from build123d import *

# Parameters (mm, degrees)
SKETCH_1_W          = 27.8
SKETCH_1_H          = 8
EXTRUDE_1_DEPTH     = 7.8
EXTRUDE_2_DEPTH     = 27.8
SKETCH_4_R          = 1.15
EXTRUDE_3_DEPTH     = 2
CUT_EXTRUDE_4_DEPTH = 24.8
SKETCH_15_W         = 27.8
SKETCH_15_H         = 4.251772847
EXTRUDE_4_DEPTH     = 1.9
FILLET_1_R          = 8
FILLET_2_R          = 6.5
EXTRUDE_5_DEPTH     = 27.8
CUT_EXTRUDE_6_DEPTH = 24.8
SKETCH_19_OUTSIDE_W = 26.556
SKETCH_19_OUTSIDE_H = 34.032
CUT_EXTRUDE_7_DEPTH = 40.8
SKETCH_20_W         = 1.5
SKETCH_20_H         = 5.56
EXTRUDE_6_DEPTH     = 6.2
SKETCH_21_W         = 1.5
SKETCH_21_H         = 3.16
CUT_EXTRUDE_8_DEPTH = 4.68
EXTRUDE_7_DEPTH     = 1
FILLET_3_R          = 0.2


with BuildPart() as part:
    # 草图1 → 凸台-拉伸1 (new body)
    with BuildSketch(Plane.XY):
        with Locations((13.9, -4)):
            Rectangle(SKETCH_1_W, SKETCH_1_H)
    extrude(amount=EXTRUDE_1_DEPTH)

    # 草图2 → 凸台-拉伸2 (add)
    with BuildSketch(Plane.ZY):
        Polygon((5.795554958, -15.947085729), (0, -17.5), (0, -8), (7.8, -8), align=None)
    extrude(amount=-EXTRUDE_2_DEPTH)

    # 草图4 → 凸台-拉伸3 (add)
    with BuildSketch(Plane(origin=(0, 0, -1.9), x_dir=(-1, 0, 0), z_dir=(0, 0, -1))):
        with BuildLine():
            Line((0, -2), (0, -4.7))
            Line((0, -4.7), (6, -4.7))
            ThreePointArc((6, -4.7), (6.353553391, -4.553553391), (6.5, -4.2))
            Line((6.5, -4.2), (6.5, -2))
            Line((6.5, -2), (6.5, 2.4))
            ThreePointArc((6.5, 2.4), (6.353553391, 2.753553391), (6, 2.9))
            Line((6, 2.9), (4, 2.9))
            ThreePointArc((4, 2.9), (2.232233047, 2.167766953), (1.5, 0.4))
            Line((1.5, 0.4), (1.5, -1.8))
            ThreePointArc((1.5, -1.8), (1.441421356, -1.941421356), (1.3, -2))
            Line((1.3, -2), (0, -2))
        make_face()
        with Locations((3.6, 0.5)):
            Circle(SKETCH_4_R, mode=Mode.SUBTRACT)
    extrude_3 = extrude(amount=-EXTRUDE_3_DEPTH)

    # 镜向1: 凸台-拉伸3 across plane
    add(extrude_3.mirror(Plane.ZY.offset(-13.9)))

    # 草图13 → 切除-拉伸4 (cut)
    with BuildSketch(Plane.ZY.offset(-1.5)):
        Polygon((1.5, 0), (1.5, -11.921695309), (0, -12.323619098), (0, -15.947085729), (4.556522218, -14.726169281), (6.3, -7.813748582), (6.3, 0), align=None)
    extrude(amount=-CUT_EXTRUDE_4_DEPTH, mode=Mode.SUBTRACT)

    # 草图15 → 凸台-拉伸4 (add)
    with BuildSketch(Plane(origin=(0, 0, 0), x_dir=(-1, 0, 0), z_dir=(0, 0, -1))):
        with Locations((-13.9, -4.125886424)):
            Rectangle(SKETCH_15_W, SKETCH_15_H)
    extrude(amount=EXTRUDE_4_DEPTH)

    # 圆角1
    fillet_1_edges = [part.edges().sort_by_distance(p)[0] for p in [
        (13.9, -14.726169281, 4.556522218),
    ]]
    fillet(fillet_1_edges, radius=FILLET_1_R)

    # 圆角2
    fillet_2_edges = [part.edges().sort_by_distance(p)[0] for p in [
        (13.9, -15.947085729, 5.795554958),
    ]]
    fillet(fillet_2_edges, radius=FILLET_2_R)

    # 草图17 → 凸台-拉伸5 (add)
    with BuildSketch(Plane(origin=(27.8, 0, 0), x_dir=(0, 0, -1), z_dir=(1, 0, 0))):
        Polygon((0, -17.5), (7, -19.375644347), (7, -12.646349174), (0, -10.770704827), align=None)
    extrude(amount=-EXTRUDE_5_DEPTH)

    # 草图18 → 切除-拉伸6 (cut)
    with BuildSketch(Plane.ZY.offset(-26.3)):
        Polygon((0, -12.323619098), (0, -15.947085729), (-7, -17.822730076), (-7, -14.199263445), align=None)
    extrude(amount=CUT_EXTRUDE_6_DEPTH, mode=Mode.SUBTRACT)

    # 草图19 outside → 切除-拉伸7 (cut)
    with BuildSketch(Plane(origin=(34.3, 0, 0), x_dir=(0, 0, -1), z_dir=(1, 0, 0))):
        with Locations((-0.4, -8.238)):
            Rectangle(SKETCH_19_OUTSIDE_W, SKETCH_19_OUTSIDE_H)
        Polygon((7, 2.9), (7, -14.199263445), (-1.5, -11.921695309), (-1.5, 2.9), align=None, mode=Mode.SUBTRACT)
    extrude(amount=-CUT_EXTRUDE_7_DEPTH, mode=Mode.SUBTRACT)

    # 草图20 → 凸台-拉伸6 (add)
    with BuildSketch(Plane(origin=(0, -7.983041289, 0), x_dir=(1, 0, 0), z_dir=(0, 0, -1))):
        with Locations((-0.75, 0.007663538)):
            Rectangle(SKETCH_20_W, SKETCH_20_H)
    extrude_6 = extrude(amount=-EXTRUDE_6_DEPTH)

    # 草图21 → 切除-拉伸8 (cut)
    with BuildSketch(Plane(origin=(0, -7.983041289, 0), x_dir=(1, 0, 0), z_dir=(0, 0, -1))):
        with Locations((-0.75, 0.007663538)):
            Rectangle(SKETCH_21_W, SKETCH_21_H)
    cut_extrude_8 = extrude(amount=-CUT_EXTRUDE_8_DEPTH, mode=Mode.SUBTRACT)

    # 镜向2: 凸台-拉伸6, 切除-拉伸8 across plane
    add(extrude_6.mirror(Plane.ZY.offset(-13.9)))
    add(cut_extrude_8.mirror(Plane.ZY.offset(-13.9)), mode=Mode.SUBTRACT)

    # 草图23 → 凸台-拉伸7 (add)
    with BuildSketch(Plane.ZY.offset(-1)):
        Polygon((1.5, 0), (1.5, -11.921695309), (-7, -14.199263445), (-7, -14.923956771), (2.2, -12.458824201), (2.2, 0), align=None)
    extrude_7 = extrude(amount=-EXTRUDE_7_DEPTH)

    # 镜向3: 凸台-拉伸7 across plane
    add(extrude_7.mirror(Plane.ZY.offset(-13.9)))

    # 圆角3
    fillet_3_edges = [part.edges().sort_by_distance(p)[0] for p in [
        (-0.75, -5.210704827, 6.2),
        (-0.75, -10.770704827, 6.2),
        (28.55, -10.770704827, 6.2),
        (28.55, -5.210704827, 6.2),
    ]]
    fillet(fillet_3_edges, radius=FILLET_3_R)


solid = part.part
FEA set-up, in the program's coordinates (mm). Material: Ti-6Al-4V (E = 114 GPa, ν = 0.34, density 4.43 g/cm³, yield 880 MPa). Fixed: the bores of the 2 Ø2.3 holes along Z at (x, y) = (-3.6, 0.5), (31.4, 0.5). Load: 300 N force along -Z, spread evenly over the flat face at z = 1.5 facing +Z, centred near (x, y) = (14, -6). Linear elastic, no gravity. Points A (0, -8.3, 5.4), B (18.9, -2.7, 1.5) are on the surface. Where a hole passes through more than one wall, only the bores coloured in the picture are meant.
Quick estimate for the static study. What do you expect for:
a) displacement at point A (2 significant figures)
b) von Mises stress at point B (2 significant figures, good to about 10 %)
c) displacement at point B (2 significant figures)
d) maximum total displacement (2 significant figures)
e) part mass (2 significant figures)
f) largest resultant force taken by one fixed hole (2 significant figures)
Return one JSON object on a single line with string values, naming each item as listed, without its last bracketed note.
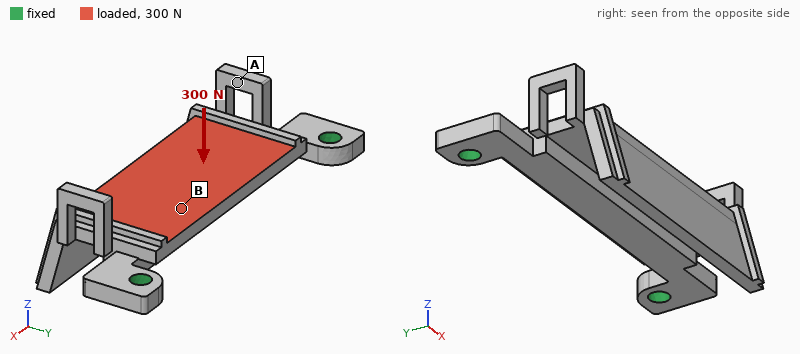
{"displacement at point A": "0.13 mm", "von Mises stress at point B": "49 MPa", "displacement at point B": "0.051 mm", "maximum total displacement": "0.21 mm", "part mass": "5.6 g", "largest resultant force taken by one fixed hole": "180 N"}
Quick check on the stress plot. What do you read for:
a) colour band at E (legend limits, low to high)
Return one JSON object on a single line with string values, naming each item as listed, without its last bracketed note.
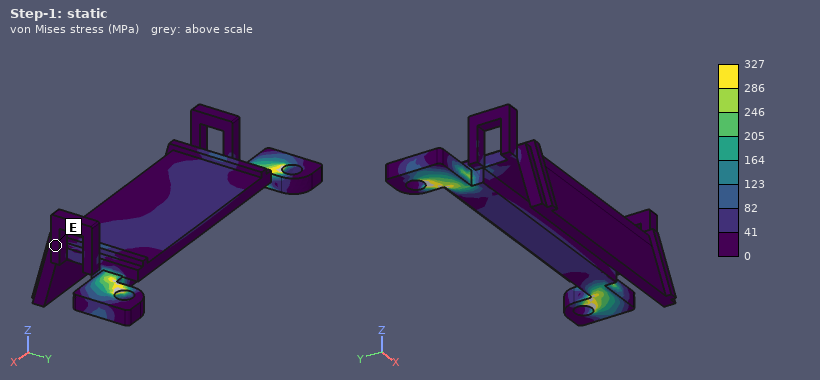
{"colour band at E": "0 to 41 MPa"}
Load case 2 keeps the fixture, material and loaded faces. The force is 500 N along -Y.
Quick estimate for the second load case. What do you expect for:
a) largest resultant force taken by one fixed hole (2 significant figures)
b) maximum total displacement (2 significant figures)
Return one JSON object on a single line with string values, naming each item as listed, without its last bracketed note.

{"largest resultant force taken by one fixed hole": "300 N", "maximum total displacement": "0.22 mm"}
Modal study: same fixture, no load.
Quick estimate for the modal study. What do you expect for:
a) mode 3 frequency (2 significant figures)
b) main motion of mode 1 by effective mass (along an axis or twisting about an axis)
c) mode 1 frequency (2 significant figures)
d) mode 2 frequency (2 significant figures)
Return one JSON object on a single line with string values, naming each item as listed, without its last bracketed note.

{"mode 3 frequency": "8900 Hz", "main motion of mode 1 by effective mass": "along Z", "mode 1 frequency": "2700 Hz", "mode 2 frequency": "7900 Hz"}
